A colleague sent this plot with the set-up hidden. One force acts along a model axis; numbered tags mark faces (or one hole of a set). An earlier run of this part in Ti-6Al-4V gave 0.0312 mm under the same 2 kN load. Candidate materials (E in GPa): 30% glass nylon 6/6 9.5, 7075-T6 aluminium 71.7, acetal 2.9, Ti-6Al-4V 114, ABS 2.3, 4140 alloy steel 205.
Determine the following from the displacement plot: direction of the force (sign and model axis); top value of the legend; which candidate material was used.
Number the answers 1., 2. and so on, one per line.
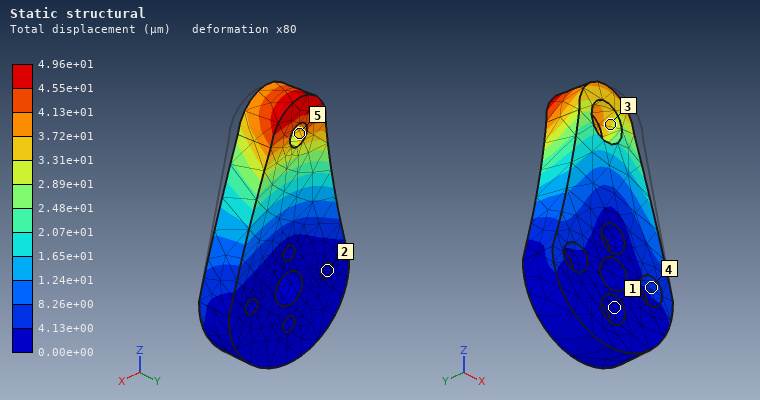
1. -X
2. 4.96e+01 µm
3. 7075-T6 aluminium
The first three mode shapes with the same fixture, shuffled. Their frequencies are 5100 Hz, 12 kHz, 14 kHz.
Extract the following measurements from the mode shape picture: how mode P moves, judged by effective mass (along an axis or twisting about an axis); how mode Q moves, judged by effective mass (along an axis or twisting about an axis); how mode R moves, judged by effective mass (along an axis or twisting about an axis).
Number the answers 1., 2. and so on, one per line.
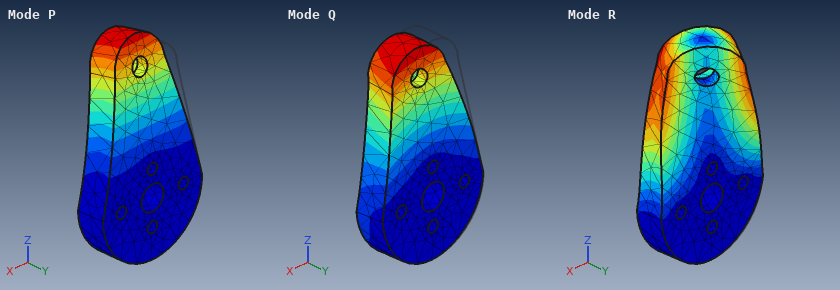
1. along Y
2. along X
3. twisting about Z
